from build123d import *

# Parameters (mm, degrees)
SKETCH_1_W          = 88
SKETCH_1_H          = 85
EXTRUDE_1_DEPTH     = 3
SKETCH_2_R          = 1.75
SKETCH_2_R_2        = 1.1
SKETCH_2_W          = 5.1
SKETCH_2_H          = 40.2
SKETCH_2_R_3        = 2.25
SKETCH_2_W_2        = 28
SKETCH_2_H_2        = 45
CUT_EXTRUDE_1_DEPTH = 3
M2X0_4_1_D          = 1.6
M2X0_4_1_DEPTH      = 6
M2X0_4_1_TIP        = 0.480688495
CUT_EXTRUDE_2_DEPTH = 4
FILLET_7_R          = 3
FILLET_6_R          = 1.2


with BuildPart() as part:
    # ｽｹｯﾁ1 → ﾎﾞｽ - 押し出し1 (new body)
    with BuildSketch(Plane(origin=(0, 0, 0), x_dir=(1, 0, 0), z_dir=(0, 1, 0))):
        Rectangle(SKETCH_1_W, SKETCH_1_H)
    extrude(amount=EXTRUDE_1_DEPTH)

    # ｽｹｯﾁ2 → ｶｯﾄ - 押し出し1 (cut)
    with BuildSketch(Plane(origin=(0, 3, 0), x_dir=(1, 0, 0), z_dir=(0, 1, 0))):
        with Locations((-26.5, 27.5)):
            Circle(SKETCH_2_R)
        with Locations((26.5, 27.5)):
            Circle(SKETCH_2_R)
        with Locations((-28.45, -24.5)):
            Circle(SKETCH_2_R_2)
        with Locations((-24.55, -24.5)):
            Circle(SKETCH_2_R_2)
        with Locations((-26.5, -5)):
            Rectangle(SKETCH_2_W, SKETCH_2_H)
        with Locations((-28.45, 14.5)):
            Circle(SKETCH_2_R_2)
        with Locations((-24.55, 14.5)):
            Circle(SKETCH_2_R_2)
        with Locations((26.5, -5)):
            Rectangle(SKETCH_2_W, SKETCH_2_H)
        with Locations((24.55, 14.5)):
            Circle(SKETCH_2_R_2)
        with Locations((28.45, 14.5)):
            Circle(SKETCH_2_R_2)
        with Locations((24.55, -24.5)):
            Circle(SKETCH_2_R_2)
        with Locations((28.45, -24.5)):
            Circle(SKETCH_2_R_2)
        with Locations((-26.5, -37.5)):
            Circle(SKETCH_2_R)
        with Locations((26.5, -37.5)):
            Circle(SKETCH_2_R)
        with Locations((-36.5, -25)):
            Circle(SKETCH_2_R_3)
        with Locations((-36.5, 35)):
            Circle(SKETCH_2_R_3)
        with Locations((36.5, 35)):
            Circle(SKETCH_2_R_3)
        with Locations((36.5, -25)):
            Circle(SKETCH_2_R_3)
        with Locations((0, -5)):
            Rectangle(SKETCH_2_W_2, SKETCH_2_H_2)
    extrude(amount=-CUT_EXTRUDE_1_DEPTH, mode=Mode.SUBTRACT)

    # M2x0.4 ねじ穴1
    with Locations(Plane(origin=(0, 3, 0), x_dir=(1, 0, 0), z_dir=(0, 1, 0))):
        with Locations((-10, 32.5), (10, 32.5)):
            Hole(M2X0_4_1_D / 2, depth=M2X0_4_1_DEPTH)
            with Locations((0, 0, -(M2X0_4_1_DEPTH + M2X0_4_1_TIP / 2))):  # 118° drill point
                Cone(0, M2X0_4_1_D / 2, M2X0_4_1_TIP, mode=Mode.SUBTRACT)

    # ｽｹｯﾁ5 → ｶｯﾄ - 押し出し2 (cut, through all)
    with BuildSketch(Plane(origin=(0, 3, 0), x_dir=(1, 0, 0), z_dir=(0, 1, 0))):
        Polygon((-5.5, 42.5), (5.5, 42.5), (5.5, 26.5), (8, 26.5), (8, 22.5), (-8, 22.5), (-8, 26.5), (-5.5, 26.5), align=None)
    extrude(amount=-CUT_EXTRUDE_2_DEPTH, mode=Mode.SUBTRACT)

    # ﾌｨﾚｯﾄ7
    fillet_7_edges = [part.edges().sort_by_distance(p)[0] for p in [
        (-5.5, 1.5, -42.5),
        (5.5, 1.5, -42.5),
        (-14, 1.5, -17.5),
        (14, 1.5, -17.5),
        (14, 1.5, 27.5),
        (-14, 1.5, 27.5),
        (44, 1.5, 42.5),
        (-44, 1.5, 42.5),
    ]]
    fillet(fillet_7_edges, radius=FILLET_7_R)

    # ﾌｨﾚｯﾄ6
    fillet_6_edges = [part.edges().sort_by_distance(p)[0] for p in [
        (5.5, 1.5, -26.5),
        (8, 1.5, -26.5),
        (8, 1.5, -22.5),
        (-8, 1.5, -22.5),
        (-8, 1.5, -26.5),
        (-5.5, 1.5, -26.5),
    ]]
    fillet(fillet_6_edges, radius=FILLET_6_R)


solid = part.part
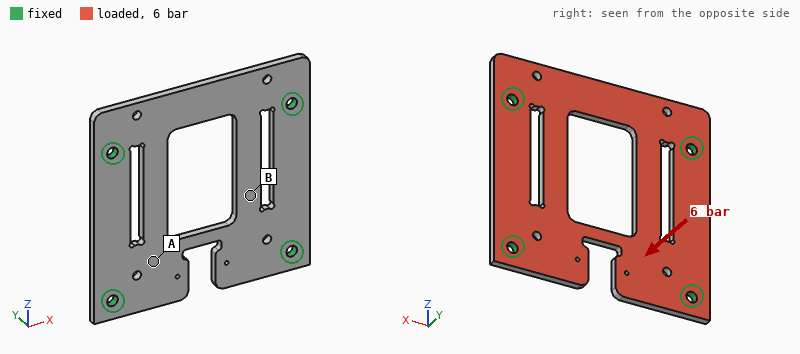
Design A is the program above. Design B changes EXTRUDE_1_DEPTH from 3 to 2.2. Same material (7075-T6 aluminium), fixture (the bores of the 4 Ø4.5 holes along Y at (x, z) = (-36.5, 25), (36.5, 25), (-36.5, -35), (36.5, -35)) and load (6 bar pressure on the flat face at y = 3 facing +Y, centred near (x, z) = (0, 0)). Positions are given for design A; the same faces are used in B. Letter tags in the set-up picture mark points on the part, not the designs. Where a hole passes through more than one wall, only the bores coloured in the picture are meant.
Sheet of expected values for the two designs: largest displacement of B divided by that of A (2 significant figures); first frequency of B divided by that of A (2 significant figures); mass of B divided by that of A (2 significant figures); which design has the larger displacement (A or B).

2.4
0.75
0.73
B
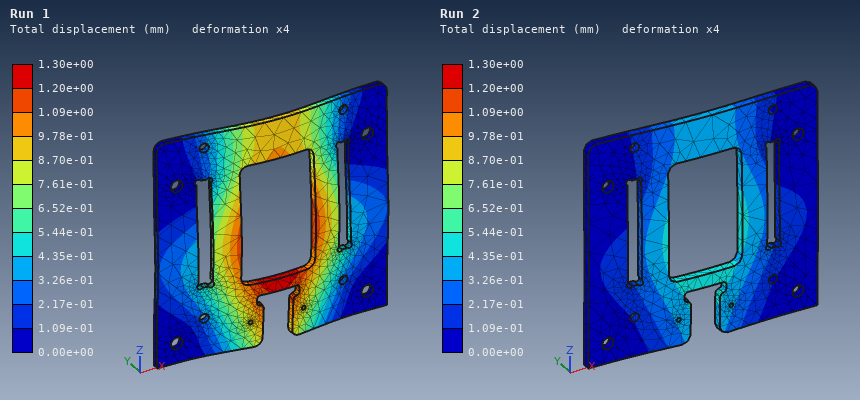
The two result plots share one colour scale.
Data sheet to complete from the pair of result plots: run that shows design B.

Run 1
